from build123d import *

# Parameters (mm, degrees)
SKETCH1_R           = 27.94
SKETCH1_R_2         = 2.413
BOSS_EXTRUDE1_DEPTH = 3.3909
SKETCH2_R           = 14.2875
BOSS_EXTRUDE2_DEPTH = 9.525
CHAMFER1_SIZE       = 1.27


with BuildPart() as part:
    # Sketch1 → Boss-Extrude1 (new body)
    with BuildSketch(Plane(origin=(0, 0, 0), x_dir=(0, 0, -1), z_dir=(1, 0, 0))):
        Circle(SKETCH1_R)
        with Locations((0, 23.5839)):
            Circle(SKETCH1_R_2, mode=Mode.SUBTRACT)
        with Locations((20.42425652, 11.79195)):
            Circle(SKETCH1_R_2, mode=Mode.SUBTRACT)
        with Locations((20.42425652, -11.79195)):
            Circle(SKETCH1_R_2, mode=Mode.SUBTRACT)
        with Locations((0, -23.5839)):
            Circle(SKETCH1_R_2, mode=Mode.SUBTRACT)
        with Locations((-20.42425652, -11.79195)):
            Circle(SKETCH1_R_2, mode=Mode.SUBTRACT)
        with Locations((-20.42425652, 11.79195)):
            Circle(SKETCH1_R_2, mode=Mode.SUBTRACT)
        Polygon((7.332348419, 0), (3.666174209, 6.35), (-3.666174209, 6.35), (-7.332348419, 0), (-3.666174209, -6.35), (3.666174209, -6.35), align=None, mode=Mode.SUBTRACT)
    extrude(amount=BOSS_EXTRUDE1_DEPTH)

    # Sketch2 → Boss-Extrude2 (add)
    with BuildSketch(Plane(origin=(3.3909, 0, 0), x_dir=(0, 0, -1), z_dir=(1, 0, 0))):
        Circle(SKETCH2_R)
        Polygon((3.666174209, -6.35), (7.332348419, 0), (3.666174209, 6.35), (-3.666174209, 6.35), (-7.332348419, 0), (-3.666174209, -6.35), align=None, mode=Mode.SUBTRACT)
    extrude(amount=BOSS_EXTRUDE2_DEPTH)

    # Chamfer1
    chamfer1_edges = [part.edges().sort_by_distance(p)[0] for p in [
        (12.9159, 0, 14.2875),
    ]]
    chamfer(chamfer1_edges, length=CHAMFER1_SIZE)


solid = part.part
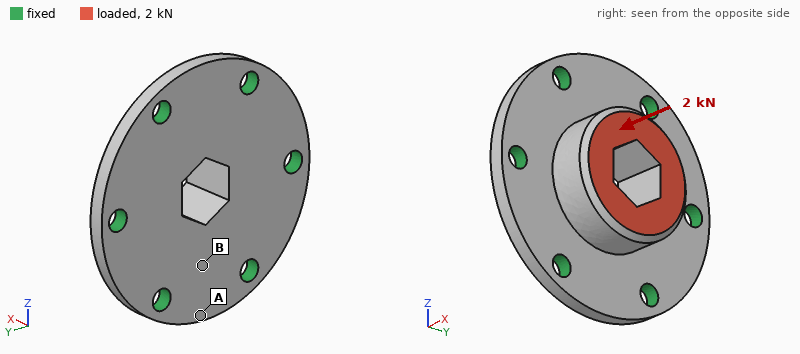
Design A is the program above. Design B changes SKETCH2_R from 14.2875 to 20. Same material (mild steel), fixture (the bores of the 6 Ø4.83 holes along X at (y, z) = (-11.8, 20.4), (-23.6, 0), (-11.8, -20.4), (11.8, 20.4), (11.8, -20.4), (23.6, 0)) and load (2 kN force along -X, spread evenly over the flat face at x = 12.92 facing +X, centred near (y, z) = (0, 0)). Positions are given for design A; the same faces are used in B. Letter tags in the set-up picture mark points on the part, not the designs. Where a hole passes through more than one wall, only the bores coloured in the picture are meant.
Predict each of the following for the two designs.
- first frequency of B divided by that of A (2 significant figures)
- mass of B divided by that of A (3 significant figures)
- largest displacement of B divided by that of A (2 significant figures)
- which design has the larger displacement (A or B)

1.5
1.48
0.28
A
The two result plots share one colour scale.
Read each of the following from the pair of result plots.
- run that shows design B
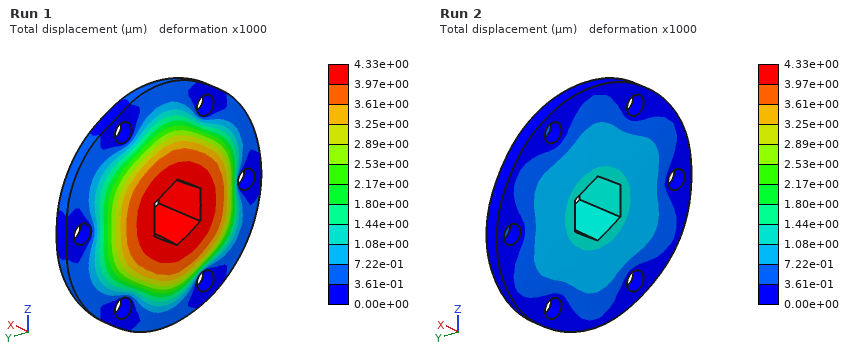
Run 2
